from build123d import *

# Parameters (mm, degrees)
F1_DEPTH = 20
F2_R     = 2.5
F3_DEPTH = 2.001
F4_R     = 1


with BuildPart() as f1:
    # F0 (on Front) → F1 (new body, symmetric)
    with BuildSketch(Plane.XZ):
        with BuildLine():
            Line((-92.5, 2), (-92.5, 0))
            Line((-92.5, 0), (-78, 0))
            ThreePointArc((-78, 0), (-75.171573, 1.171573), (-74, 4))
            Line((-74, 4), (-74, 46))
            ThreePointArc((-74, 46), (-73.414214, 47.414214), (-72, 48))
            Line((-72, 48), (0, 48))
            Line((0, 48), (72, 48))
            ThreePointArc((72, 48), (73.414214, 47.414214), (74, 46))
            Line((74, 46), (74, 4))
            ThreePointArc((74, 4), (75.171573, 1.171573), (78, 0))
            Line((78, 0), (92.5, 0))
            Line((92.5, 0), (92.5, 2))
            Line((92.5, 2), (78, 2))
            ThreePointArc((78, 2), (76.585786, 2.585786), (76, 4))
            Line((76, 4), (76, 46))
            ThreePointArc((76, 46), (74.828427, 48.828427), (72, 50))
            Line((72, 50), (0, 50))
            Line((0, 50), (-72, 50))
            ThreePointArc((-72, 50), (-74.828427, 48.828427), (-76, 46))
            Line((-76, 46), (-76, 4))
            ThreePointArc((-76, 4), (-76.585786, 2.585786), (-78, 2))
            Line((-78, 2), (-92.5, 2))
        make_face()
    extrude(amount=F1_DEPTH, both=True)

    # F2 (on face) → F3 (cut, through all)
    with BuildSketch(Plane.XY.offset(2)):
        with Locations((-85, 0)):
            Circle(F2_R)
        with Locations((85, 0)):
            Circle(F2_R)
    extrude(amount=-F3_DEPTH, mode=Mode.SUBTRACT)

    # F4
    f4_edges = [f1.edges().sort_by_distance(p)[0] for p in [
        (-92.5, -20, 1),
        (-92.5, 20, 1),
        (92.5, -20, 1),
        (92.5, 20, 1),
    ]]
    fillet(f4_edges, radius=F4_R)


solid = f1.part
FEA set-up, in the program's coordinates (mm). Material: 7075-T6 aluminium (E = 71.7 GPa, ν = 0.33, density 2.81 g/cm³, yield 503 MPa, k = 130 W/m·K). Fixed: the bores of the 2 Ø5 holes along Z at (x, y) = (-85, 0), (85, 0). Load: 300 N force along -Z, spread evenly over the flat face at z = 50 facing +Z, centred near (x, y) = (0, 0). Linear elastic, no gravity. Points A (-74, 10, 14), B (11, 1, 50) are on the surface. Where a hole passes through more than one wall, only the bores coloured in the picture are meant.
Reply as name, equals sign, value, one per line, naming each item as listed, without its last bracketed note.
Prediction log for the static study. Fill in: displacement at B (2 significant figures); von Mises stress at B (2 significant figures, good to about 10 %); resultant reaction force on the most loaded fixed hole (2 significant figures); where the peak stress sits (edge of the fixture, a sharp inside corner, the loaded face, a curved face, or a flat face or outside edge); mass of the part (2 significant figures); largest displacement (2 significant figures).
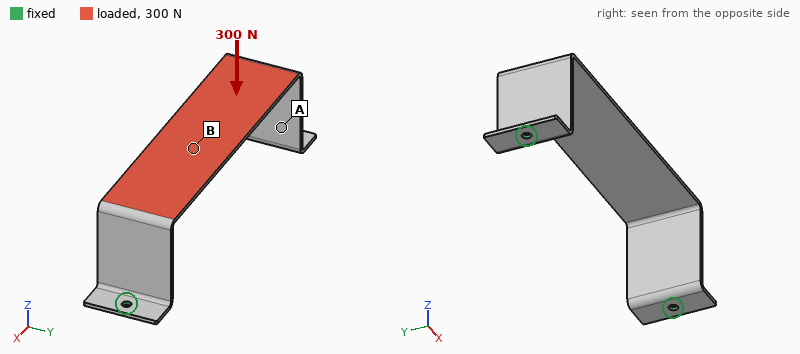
displacement at B = 2.0 mm
von Mises stress at B = 84 MPa
resultant reaction force on the most loaded fixed hole = 180 N
where the peak stress sits = a curved face
mass of the part = 62 g
largest displacement = 2.1 mm
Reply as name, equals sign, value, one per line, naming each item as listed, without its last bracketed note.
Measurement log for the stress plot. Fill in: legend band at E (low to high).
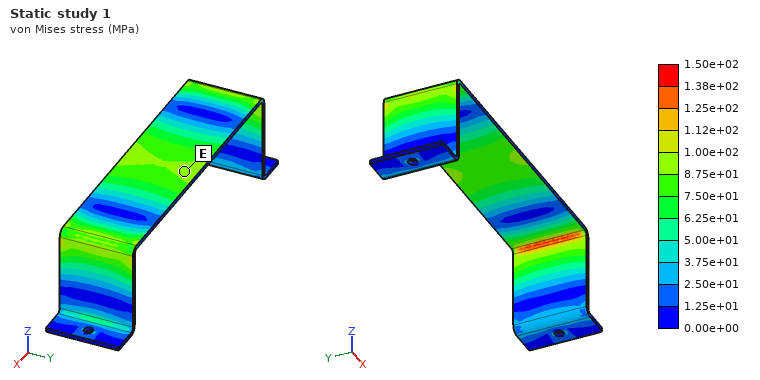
legend band at E = 8.75e+01 to 1.00e+02 MPa
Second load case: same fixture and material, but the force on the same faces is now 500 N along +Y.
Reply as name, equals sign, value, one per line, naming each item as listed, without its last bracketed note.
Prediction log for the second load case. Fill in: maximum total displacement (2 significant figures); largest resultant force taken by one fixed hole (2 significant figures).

maximum total displacement = 2.0 mm
largest resultant force taken by one fixed hole = 250 N
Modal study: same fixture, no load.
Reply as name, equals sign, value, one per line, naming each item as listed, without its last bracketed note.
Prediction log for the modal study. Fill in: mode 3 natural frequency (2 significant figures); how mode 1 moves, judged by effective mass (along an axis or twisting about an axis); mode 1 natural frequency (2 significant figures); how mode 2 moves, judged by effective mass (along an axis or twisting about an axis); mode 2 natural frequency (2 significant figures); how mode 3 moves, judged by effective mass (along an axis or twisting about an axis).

mode 3 natural frequency = 410 Hz
how mode 1 moves, judged by effective mass = along X
mode 1 natural frequency = 300 Hz
how mode 2 moves, judged by effective mass = along Z
mode 2 natural frequency = 380 Hz
how mode 3 moves, judged by effective mass = along Y
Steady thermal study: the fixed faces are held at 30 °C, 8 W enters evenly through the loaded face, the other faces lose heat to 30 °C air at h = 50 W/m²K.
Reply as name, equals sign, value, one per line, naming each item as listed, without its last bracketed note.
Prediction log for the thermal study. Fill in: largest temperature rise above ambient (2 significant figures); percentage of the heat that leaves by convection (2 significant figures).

largest temperature rise above ambient = 15 K
percentage of the heat that leaves by convection = 75 %
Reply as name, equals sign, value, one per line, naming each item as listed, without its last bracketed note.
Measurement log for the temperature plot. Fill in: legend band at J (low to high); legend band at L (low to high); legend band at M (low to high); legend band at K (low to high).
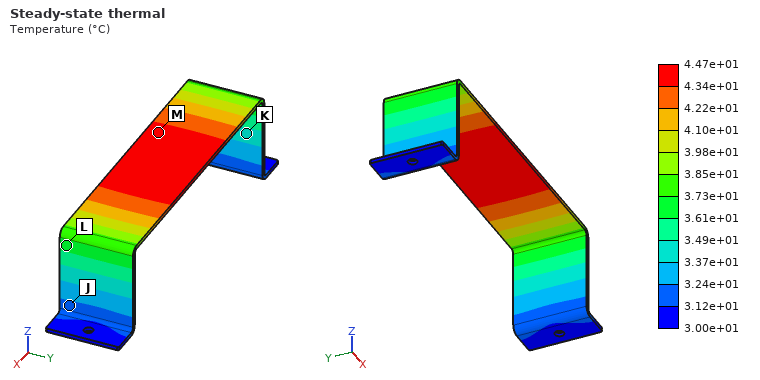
legend band at J = 3.12e+01 to 3.24e+01 °C
legend band at L = 3.61e+01 to 3.73e+01 °C
legend band at M = 4.34e+01 to 4.47e+01 °C
legend band at K = 3.37e+01 to 3.49e+01 °C
